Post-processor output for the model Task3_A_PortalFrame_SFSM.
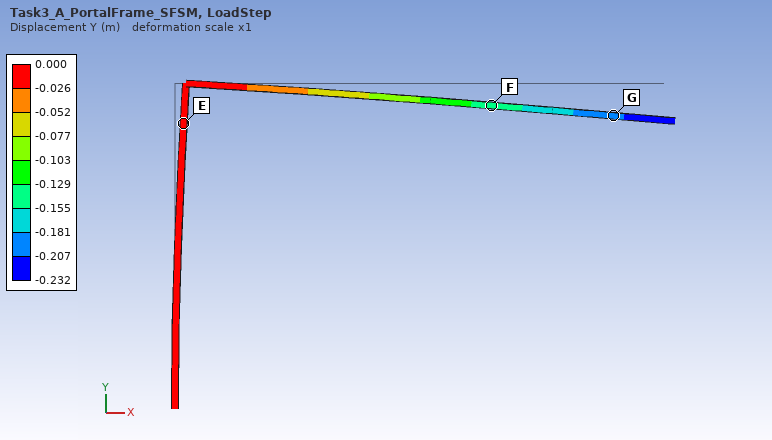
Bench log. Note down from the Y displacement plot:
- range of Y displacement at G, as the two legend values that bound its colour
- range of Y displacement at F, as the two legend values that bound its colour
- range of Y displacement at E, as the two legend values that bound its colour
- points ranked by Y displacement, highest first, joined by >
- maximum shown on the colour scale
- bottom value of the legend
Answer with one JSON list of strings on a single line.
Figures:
["-0.207 to -0.181 m", "-0.155 to -0.129 m", "-0.026 to 0.000 m", "E > F > G", "0.000 m", "-0.232 m"]
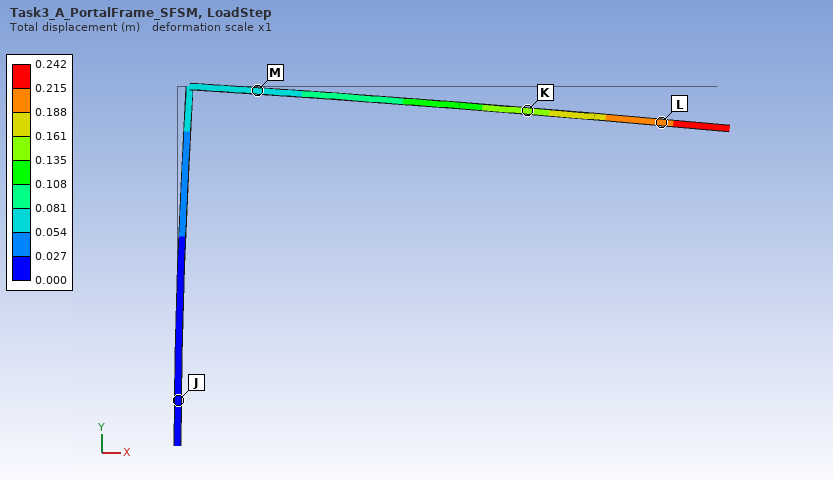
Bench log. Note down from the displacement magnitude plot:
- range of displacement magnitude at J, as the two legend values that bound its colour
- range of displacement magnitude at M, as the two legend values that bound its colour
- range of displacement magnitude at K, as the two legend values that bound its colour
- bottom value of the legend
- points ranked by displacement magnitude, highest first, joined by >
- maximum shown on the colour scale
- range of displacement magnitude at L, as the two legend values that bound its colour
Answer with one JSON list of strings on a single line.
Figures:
["0.000 to 0.027 m", "0.054 to 0.081 m", "0.135 to 0.161 m", "0.000 m", "L > K > M > J", "0.242 m", "0.188 to 0.215 m"]
